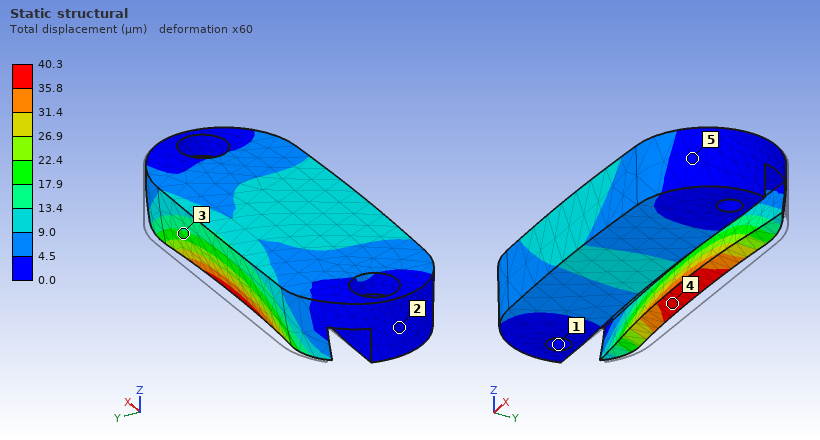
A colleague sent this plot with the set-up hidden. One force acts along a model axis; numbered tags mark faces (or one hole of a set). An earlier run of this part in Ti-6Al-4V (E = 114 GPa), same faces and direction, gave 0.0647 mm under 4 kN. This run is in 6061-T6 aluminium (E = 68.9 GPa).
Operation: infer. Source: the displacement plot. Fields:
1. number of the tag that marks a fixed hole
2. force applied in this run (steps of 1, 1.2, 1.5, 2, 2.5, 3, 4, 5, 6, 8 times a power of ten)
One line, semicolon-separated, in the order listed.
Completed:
1; 1.5 kN
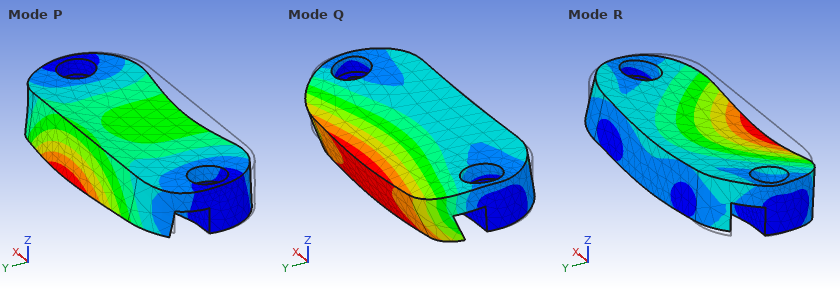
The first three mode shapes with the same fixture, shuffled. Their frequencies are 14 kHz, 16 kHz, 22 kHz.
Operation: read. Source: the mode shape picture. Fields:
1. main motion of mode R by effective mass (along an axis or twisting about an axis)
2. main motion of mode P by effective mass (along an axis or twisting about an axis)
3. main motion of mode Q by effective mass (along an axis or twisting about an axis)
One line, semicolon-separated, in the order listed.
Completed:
along Z; along Y; along Z
